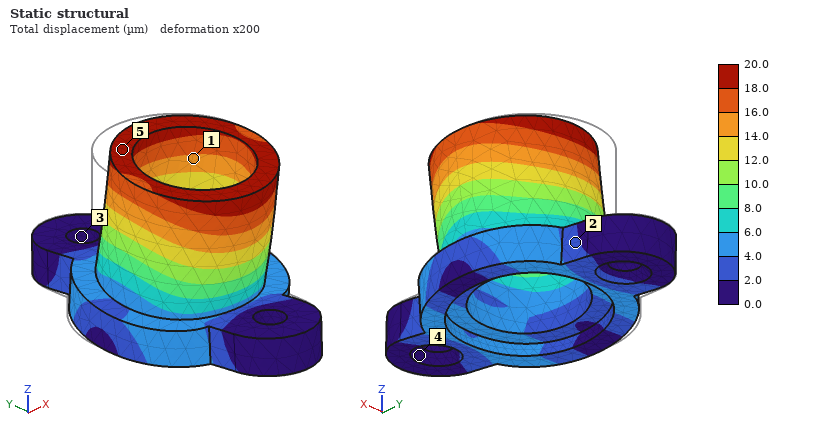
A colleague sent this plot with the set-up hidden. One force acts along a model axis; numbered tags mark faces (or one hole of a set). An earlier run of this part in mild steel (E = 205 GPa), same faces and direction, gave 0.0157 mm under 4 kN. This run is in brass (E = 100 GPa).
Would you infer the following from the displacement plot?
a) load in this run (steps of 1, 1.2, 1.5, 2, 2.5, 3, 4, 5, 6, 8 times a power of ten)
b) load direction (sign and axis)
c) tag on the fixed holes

2.5 kN
-Y
3
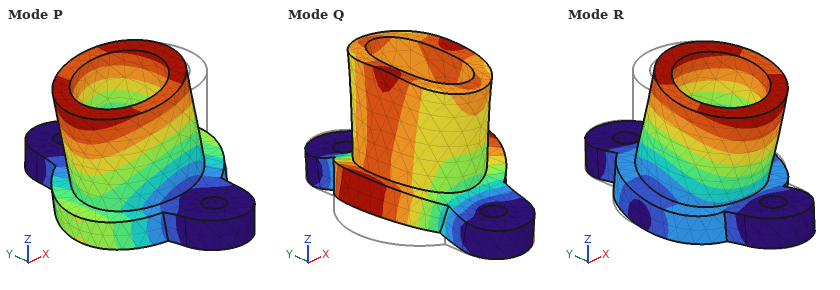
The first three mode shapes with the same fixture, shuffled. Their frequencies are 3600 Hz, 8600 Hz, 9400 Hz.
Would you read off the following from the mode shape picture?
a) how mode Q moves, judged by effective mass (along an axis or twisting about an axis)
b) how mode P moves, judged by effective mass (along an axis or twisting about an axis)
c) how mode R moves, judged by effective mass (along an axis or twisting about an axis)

along Z
along X
along Y
